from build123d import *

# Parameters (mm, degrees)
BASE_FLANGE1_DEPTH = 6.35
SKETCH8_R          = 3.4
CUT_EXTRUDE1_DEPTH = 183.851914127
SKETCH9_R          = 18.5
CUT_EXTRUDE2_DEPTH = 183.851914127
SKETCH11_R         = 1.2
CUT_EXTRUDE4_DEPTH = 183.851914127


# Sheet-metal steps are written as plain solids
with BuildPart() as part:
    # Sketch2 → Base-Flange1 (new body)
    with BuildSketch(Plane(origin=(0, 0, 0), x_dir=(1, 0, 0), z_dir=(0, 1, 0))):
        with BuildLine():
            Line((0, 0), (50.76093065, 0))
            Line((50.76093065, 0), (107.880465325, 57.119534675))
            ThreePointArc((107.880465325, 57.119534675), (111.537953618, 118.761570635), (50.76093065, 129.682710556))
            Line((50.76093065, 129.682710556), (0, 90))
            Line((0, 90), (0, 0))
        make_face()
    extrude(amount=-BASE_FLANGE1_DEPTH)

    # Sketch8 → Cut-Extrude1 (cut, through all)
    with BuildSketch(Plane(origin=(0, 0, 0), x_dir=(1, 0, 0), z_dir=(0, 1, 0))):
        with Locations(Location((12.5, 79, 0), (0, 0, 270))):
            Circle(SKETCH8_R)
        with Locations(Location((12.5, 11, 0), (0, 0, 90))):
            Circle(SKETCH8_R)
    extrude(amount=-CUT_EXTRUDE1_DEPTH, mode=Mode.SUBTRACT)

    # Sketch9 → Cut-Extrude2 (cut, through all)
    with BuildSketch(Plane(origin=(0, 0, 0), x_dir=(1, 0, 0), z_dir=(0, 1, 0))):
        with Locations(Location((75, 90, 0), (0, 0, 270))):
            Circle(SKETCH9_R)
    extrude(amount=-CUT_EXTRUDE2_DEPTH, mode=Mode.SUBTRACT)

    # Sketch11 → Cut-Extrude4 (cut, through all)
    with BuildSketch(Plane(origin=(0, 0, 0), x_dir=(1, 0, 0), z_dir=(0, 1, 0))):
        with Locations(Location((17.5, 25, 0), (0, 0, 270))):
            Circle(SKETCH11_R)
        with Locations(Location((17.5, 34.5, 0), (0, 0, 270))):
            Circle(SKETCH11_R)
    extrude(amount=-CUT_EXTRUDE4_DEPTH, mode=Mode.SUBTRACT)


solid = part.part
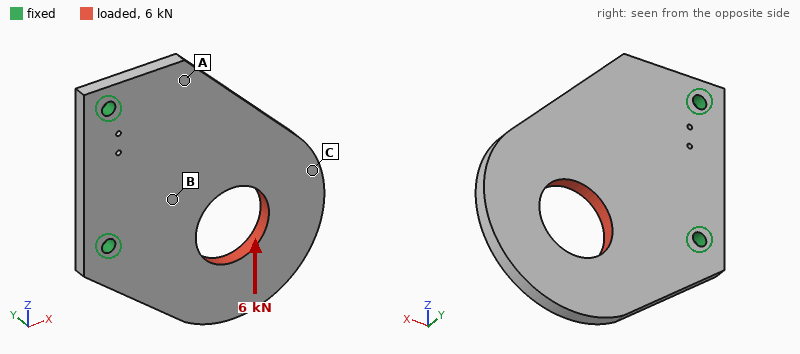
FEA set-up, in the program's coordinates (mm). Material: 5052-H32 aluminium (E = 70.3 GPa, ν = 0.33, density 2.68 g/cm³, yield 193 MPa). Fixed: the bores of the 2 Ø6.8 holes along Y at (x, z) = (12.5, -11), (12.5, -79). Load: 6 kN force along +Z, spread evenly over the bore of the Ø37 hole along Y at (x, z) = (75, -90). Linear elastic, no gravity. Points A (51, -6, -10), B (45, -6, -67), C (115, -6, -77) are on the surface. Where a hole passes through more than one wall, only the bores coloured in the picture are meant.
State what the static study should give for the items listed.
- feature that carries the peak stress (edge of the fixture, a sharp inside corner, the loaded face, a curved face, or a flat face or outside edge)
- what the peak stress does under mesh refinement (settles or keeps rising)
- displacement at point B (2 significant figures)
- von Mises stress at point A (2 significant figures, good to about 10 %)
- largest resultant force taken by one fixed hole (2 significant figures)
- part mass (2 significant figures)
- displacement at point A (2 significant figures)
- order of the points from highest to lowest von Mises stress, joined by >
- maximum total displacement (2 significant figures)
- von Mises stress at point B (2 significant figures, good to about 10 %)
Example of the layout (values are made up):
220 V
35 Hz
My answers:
edge of the fixture
keeps rising
0.026 mm
18 MPa
6.1 kN
190 g
0.030 mm
B > A > C
0.10 mm
29 MPa
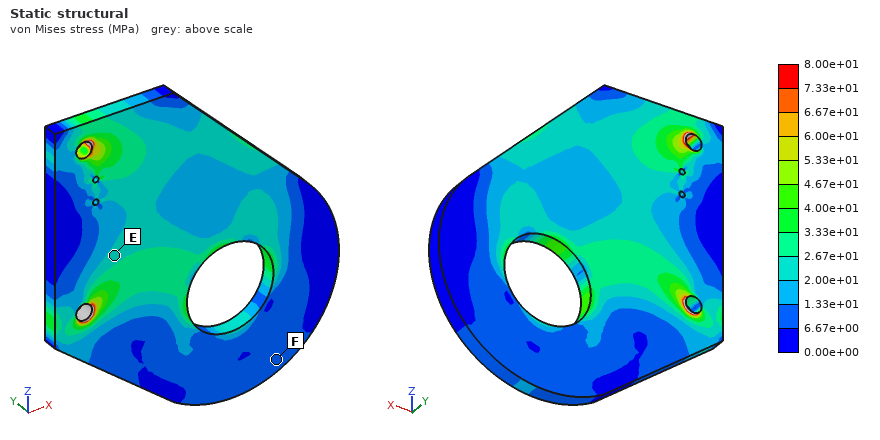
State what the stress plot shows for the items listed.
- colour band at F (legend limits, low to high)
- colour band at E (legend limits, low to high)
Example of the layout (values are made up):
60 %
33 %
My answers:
6.67e+00 to 1.33e+01 MPa
2.00e+01 to 2.67e+01 MPa
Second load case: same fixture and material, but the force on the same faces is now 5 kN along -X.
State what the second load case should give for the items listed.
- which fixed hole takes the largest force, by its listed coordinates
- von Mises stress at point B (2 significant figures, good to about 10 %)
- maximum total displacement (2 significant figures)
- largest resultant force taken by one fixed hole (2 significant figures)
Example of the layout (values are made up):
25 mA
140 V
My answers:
(12.5, -79)
18 MPa
55 µm
5.7 kN
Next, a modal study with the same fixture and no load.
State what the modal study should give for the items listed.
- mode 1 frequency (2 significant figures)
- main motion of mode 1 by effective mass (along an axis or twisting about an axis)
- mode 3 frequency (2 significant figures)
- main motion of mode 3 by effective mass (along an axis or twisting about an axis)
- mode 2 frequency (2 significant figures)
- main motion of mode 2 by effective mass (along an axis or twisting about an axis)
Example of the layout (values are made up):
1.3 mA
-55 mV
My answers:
480 Hz
along Y
2200 Hz
along Y
1100 Hz
twisting about X
